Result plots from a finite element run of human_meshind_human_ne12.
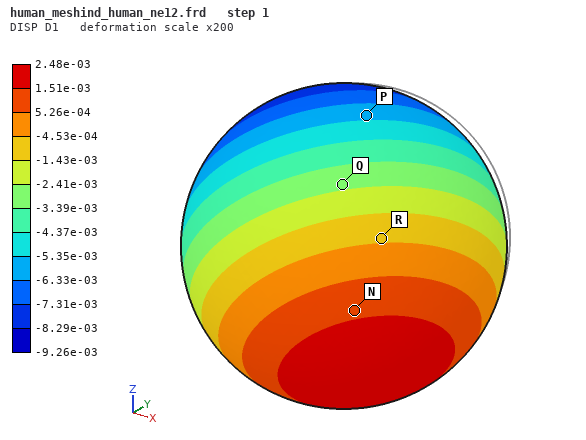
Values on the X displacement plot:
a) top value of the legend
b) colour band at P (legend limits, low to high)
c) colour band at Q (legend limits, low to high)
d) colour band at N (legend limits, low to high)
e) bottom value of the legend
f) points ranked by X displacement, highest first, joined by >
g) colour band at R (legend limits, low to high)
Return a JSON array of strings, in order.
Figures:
["2.48e-03", "-6.33e-03 to -5.35e-03", "-3.39e-03 to -2.41e-03", "5.26e-04 to 1.51e-03", "-9.26e-03", "N > R > Q > P", "-1.43e-03 to -4.53e-04"]
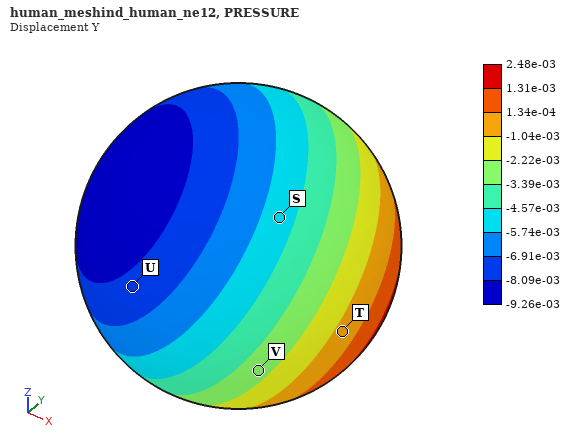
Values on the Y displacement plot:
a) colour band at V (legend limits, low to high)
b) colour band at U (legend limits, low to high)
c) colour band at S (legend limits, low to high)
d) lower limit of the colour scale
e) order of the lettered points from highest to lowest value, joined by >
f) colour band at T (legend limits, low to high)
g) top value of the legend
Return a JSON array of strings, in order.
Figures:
["-3.39e-03 to -2.22e-03", "-8.09e-03 to -6.91e-03", "-5.74e-03 to -4.57e-03", "-9.26e-03", "T > V > S > U", "-1.04e-03 to 1.34e-04", "2.48e-03"]
